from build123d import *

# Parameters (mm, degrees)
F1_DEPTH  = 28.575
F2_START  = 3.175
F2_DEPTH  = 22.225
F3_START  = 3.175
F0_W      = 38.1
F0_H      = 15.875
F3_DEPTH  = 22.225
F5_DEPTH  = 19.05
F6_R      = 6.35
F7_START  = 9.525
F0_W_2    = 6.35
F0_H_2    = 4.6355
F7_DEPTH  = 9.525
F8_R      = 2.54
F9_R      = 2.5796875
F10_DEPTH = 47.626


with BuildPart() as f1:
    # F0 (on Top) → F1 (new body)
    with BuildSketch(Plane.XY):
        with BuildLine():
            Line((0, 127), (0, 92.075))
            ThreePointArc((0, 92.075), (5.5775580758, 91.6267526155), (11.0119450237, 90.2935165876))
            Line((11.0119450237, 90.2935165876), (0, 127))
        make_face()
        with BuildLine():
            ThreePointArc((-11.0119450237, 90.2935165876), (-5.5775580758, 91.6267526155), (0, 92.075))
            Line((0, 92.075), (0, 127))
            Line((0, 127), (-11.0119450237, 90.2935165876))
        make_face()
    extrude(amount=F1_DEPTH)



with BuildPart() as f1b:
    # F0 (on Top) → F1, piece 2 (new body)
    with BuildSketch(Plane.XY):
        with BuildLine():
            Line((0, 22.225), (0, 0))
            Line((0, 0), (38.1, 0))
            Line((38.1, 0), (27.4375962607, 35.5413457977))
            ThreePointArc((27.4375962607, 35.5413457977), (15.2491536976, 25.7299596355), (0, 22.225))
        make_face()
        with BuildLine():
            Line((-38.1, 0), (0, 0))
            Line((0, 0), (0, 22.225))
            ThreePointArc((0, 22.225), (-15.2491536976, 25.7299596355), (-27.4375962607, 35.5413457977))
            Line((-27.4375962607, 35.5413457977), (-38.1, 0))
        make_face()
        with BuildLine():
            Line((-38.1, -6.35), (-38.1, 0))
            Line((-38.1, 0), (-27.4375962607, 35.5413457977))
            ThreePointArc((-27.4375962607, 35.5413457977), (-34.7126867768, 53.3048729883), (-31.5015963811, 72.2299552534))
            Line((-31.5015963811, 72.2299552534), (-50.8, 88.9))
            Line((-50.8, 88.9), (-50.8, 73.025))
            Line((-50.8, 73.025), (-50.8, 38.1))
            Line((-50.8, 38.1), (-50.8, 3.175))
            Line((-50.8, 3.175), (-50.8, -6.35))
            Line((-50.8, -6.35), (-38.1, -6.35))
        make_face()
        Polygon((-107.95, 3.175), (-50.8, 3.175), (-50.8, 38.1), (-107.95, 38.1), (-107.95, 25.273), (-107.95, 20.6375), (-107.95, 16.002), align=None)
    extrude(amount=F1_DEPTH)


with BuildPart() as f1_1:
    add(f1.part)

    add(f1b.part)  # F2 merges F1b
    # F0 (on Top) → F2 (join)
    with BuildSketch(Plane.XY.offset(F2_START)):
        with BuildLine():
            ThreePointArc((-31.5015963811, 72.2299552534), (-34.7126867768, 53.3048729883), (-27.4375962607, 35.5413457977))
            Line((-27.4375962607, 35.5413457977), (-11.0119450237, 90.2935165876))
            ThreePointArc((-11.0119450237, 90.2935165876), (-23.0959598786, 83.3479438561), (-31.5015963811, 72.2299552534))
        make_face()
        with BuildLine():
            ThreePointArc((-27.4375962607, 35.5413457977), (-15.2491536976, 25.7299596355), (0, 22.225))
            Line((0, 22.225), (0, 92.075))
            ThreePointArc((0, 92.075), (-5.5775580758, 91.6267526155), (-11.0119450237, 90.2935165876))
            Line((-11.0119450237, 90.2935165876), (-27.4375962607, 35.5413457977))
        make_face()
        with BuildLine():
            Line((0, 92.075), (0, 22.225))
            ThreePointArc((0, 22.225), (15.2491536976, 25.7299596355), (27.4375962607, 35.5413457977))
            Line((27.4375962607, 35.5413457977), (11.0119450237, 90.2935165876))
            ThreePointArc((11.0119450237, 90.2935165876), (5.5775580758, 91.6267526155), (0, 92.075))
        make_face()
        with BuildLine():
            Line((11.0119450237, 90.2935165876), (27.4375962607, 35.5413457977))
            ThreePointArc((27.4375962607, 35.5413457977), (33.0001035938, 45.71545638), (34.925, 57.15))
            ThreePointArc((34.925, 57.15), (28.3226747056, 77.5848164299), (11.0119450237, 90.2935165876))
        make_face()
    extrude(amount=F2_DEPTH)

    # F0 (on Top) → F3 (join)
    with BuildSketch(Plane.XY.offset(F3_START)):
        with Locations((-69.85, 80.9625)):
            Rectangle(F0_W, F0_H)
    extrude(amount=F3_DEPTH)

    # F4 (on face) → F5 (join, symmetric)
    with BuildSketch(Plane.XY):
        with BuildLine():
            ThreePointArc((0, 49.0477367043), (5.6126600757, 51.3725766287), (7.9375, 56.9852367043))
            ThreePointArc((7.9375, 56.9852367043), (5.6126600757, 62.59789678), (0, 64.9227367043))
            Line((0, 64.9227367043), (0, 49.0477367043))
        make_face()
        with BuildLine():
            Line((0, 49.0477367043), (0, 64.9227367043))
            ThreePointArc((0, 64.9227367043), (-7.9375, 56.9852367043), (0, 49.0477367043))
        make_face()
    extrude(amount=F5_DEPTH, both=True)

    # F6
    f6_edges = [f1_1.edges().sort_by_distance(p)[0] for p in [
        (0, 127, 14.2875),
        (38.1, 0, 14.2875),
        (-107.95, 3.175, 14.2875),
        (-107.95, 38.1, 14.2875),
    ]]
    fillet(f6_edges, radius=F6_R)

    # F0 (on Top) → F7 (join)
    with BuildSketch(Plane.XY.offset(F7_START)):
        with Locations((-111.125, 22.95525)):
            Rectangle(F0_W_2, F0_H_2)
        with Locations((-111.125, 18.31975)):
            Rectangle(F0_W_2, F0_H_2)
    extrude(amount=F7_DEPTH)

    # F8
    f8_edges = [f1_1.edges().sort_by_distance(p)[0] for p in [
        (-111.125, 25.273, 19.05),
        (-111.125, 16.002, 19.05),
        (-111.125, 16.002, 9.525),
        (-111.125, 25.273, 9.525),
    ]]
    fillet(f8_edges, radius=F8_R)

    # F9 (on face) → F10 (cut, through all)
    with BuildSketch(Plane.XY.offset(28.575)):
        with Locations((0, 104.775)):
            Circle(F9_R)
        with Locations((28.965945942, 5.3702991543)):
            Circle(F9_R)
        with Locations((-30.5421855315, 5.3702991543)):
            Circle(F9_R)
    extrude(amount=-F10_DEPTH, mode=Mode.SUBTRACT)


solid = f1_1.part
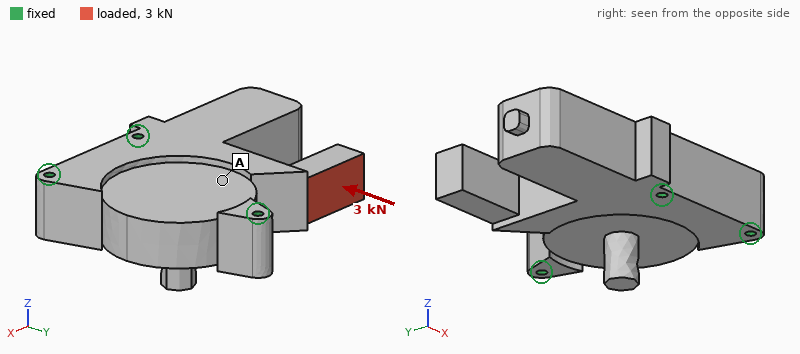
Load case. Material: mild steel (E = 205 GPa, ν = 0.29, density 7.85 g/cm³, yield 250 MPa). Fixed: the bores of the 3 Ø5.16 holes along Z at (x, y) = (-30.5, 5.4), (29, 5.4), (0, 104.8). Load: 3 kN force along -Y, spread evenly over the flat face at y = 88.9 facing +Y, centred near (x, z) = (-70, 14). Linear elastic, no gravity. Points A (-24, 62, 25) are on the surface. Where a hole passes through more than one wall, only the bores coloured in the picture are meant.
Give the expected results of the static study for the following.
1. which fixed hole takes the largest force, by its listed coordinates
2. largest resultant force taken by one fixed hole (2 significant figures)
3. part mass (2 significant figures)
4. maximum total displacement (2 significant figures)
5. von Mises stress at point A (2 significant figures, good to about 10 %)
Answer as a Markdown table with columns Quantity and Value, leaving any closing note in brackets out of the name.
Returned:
| Quantity | Value |
|---|---|
| which fixed hole takes the largest force, by its listed coordinates | (-30.5, 5.4) |
| largest resultant force taken by one fixed hole | 3.4 kN |
| part mass | 2.1 kg |
| maximum total displacement | 71 µm |
| von Mises stress at point A | 8.4 MPa |
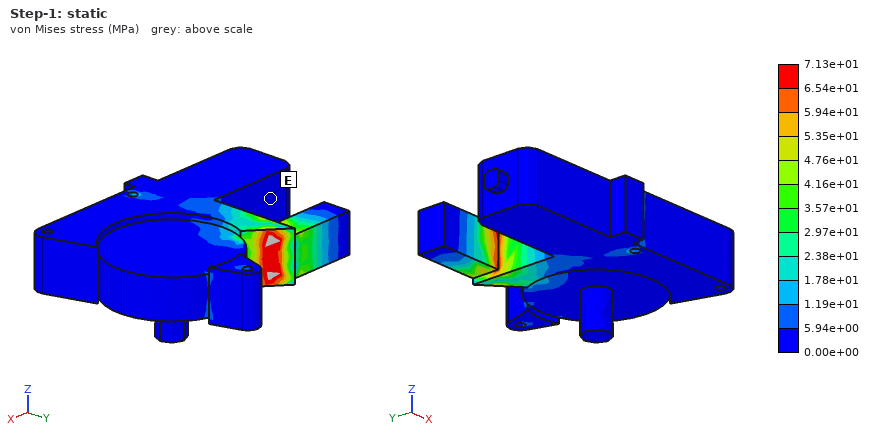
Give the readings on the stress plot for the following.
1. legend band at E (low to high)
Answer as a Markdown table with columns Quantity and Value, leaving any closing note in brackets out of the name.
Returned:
| Quantity | Value |
|---|---|
| legend band at E | 0.00e+00 to 5.94e+00 MPa |
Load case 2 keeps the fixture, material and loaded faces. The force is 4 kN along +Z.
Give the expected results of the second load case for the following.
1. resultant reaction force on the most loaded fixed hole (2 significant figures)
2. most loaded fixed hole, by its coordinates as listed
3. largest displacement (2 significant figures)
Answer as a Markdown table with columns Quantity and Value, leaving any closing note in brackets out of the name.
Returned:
| Quantity | Value |
|---|---|
| resultant reaction force on the most loaded fixed hole | 3.4 kN |
| most loaded fixed hole, by its coordinates as listed | (-30.5, 5.4) |
| largest displacement | 0.11 mm |
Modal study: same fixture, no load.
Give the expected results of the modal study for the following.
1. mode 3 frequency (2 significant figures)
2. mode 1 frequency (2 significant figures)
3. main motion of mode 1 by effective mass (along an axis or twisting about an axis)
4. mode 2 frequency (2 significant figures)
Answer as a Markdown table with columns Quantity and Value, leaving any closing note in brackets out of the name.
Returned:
| Quantity | Value |
|---|---|
| mode 3 frequency | 3700 Hz |
| mode 1 frequency | 2800 Hz |
| main motion of mode 1 by effective mass | along Z |
| mode 2 frequency | 3700 Hz |
